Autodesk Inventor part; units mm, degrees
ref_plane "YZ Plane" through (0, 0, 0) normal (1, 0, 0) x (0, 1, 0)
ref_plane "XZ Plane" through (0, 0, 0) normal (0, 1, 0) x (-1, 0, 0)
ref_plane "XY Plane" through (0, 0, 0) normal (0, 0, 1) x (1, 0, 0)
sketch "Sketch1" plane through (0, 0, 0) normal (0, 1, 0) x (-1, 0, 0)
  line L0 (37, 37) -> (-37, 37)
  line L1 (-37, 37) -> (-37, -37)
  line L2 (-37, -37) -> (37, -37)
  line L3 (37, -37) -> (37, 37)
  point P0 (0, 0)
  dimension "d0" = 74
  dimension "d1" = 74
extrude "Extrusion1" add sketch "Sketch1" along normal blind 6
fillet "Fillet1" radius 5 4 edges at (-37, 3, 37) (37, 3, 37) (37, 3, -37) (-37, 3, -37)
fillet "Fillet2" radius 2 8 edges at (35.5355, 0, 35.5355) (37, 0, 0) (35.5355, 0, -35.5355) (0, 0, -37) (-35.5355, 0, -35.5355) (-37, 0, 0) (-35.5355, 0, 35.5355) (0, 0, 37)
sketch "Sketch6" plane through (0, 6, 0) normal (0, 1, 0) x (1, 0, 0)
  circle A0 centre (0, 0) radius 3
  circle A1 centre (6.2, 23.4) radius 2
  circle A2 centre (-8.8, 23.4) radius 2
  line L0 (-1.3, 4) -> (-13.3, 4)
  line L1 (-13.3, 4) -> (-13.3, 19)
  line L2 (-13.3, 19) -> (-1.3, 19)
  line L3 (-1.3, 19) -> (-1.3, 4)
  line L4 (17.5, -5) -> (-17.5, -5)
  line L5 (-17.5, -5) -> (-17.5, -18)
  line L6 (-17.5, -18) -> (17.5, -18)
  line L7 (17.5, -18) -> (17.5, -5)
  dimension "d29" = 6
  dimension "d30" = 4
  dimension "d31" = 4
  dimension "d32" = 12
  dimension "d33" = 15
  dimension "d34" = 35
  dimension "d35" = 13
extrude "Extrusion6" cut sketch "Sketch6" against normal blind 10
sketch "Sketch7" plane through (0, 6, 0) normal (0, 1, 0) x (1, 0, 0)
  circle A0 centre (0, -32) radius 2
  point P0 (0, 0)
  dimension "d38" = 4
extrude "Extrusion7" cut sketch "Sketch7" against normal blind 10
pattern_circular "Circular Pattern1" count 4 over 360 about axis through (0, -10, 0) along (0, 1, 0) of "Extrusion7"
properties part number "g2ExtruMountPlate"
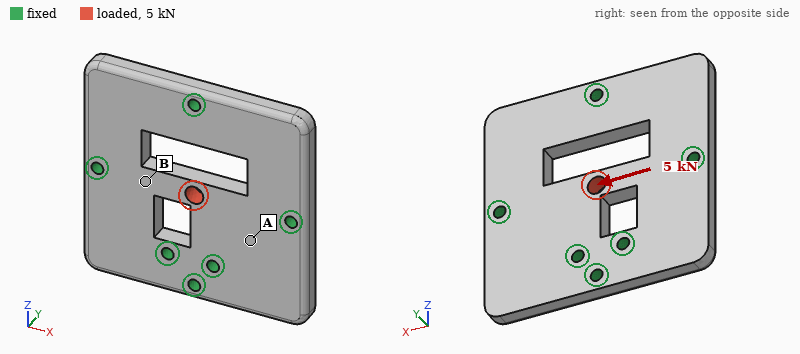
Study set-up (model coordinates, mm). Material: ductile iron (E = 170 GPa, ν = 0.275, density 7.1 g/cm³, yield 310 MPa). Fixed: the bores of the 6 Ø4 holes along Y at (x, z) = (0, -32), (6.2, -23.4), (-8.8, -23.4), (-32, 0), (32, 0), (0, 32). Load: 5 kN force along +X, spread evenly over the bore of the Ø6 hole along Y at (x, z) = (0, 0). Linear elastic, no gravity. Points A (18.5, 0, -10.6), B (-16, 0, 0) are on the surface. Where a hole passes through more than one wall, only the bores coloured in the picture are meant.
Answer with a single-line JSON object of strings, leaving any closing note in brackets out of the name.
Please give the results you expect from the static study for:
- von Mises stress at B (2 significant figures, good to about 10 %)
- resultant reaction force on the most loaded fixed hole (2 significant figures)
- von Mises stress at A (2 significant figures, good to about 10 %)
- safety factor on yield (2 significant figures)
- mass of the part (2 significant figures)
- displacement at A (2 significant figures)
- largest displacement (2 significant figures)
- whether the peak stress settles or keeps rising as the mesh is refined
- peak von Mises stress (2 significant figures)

{"von Mises stress at B": "30 MPa", "resultant reaction force on the most loaded fixed hole": "1.9 kN", "von Mises stress at A": "11 MPa", "safety factor on yield": "3.6", "mass of the part": "200 g", "displacement at A": "1.8 µm", "largest displacement": "6.4 µm", "whether the peak stress settles or keeps rising as the mesh is refined": "settles", "peak von Mises stress": "87 MPa"}
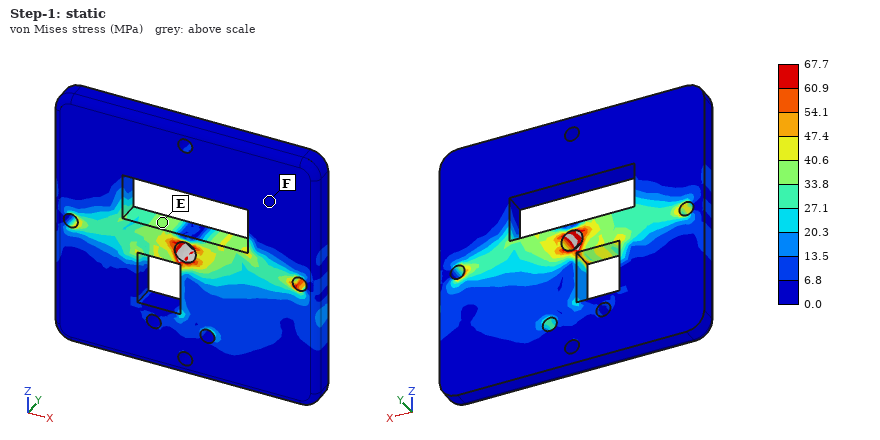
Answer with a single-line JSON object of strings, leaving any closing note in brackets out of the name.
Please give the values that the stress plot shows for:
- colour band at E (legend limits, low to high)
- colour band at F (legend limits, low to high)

{"colour band at E": "33.8 to 40.6 MPa", "colour band at F": "0.0 to 6.8 MPa"}
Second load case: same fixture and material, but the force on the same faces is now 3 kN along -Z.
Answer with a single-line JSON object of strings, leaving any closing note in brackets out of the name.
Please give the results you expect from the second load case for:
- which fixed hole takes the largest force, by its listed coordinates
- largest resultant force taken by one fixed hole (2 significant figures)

{"which fixed hole takes the largest force, by its listed coordinates": "(6.2, -23.4)", "largest resultant force taken by one fixed hole": "1.7 kN"}
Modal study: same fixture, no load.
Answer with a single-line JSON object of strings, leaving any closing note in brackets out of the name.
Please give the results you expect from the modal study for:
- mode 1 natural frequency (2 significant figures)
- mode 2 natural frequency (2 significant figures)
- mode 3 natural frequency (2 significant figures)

{"mode 1 natural frequency": "6300 Hz", "mode 2 natural frequency": "6500 Hz", "mode 3 natural frequency": "7600 Hz"}
